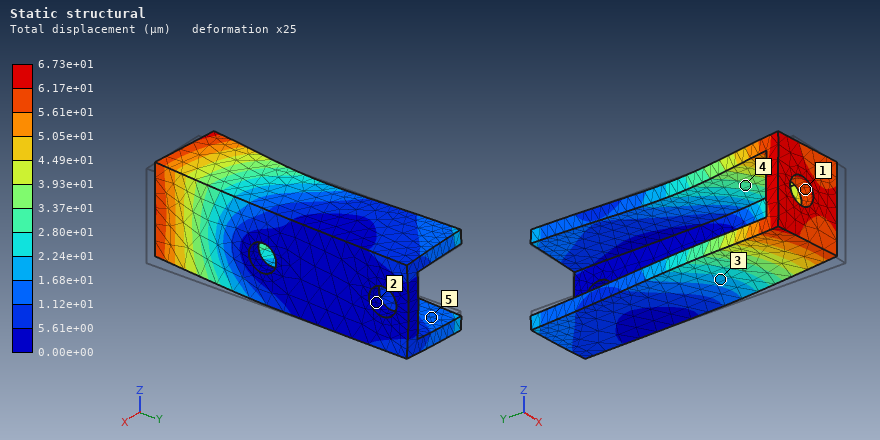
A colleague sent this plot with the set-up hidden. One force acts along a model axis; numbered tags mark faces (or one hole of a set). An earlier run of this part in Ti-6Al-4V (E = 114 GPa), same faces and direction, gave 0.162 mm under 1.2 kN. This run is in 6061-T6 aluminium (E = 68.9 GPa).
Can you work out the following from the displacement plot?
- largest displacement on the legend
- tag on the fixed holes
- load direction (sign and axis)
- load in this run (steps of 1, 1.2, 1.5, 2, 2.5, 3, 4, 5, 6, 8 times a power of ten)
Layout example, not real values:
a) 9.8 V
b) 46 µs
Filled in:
a) 6.73e+01 µm
b) 2
c) -X
d) 300 N
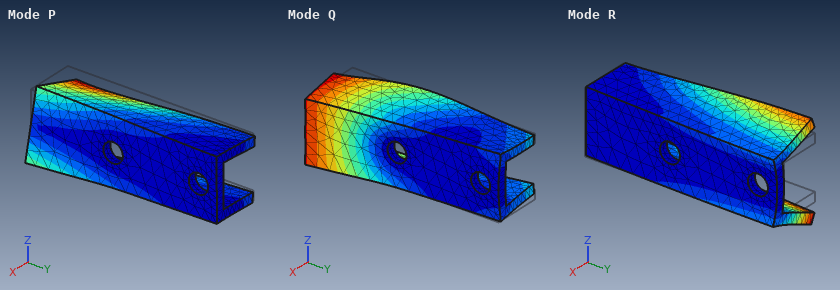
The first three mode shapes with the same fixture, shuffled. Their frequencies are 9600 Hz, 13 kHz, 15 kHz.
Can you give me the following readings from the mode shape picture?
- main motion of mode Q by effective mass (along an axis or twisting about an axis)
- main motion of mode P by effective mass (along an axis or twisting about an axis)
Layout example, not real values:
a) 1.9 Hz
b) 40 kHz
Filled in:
a) along X
b) along Z
